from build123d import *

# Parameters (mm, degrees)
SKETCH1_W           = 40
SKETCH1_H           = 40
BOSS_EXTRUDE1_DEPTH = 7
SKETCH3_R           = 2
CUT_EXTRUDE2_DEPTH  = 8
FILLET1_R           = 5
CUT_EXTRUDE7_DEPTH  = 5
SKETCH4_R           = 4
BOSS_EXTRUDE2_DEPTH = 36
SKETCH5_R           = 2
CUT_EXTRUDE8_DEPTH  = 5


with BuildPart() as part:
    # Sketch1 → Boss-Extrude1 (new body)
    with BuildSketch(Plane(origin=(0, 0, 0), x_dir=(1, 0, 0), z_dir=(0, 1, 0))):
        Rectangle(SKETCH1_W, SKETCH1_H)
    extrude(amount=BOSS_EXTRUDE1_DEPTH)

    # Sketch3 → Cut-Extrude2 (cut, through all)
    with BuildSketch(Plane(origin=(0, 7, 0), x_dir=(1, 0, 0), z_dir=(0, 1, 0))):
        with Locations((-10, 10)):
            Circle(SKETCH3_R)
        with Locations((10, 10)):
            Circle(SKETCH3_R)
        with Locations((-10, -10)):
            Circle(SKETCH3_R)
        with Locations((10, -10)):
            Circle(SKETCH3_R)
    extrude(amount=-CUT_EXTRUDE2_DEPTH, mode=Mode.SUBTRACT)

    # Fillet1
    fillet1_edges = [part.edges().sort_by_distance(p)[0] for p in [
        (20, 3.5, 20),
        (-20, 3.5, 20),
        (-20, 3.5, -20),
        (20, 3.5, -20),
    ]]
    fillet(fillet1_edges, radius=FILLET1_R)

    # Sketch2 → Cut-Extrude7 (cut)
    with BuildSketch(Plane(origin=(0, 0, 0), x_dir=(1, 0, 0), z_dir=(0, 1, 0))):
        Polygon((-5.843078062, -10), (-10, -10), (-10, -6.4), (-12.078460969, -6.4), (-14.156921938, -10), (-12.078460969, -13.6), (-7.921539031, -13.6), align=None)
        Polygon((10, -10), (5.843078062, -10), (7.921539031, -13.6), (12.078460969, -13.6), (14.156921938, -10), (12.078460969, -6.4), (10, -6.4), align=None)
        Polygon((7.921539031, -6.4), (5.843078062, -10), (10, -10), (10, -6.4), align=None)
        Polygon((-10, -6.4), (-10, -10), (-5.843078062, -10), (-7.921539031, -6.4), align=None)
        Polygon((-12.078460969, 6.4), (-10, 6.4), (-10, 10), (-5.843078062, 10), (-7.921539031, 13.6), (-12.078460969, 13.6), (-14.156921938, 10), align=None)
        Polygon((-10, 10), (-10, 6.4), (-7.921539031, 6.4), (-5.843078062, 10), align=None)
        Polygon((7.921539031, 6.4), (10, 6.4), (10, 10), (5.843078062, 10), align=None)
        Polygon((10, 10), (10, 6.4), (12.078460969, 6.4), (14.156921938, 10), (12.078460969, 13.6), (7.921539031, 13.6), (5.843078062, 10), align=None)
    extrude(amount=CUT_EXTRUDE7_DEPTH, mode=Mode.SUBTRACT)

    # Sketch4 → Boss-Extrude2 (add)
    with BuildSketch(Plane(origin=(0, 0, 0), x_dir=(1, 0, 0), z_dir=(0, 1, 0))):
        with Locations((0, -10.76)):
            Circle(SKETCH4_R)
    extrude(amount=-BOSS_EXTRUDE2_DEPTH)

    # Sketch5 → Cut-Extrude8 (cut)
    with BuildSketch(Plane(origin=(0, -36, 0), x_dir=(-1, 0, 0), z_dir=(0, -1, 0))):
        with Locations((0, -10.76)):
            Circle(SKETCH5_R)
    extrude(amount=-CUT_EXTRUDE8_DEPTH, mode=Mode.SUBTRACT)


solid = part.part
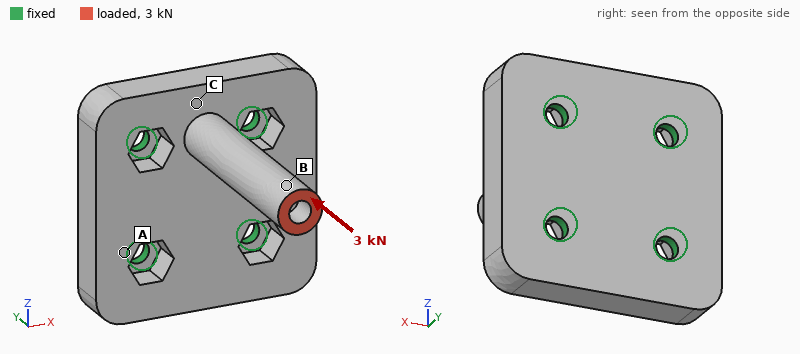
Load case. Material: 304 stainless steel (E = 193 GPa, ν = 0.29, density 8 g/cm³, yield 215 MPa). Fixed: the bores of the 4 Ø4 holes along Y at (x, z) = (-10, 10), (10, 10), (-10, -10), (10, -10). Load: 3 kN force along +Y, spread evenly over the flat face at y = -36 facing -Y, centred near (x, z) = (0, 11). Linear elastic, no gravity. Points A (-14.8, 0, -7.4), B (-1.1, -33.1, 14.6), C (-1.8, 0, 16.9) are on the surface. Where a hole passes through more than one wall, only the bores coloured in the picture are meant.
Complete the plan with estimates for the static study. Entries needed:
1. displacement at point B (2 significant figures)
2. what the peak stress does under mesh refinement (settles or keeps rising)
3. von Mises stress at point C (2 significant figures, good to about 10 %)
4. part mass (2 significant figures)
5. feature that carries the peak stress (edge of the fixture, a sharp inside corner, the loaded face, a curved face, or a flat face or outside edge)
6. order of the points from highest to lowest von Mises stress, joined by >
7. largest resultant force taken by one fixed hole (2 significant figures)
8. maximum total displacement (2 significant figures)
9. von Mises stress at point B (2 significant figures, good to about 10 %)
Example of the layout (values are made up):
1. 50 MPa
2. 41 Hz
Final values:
1. 21 µm
2. keeps rising
3. 40 MPa
4. 94 g
5. edge of the fixture
6. B > C > A
7. 1.6 kN
8. 22 µm
9. 77 MPa
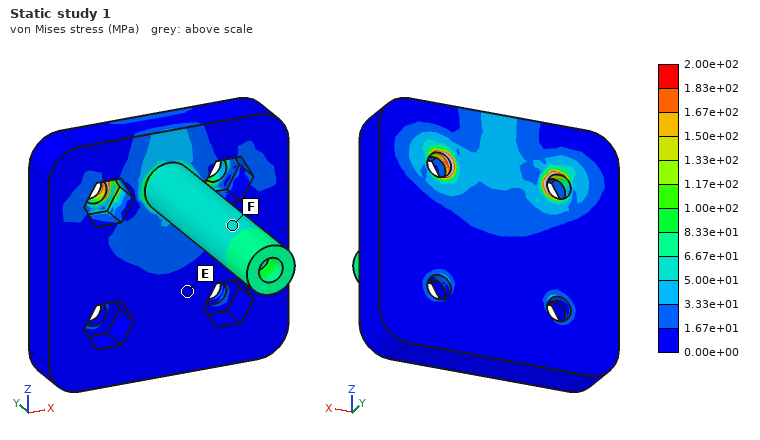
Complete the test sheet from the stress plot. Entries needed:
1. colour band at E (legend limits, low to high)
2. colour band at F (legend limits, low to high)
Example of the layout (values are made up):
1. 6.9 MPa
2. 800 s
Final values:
1. 0.00e+00 to 1.67e+01 MPa
2. 5.00e+01 to 6.67e+01 MPa
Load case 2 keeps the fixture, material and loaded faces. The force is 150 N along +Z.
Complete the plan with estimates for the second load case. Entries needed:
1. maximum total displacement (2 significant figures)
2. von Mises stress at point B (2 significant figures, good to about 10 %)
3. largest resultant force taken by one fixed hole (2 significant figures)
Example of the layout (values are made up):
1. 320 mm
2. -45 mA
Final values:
1. 81 µm
2. 11 MPa
3. 230 N
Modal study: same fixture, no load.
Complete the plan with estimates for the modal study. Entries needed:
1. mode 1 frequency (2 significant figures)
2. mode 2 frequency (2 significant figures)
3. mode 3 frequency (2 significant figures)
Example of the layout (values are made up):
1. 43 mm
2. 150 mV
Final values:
1. 3700 Hz
2. 3800 Hz
3. 17 kHz
